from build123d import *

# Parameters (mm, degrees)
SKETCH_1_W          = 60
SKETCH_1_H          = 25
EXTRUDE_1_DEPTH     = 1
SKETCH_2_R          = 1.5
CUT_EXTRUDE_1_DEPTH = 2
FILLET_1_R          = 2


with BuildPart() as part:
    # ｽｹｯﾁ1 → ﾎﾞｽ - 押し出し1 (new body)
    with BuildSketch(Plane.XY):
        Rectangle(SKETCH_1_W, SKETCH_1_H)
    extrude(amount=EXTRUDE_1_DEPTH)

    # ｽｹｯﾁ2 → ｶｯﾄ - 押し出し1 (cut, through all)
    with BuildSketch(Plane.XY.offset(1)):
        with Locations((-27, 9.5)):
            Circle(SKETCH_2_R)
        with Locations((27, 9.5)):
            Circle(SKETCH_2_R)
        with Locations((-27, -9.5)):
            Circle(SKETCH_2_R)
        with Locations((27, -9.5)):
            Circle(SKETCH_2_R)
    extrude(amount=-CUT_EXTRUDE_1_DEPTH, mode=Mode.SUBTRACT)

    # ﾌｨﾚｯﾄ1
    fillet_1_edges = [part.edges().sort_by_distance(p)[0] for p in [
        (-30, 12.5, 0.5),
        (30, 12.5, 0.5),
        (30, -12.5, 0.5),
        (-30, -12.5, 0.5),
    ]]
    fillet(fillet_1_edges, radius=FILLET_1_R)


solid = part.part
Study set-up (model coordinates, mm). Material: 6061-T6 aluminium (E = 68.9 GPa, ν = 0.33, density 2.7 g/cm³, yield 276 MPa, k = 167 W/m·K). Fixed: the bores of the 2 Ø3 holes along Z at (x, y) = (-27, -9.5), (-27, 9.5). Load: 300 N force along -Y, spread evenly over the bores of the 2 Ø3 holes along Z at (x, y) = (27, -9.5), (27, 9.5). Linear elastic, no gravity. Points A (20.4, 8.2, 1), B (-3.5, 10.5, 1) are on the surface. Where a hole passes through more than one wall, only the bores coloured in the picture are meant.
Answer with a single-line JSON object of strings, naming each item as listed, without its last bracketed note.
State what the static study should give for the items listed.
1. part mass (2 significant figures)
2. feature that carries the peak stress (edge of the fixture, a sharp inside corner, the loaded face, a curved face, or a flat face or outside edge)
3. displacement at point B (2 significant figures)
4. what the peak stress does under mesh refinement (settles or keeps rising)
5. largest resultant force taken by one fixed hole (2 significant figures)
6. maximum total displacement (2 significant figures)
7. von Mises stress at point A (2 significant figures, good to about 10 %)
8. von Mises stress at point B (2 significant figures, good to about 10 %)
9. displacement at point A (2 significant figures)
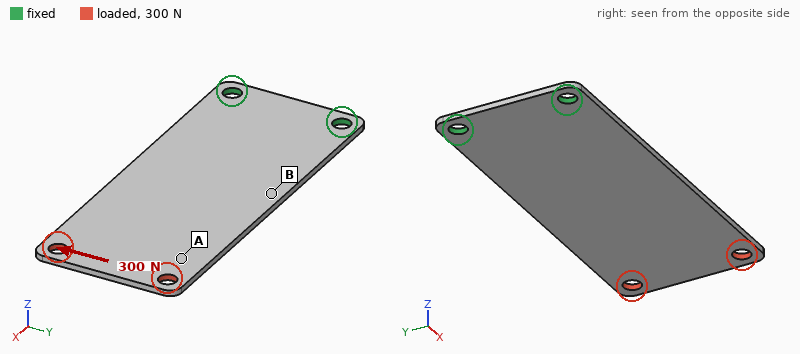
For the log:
{"part mass": "4.0 g", "feature that carries the peak stress": "edge of the fixture", "displacement at point B": "0.065 mm", "what the peak stress does under mesh refinement": "keeps rising", "largest resultant force taken by one fixed hole": "830 N", "maximum total displacement": "0.23 mm", "von Mises stress at point A": "22 MPa", "von Mises stress at point B": "74 MPa", "displacement at point A": "0.17 mm"}
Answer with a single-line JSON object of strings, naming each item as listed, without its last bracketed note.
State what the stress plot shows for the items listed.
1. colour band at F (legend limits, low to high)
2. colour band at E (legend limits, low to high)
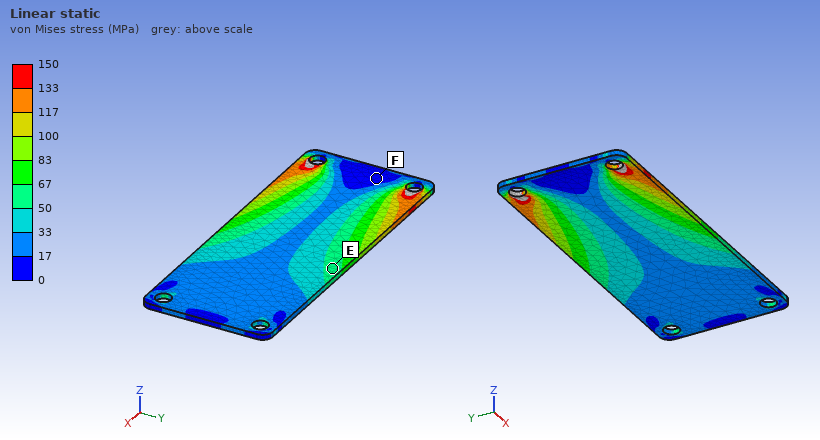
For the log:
{"colour band at F": "0 to 17 MPa", "colour band at E": "50 to 67 MPa"}
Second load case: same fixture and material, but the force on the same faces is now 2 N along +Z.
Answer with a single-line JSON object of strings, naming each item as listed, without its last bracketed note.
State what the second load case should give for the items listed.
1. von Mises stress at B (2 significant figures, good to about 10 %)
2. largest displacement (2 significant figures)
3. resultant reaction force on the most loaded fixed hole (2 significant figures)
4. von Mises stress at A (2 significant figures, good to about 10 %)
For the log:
{"von Mises stress at B": "15 MPa", "largest displacement": "0.77 mm", "resultant reaction force on the most loaded fixed hole": "1.0 N", "von Mises stress at A": "3.6 MPa"}
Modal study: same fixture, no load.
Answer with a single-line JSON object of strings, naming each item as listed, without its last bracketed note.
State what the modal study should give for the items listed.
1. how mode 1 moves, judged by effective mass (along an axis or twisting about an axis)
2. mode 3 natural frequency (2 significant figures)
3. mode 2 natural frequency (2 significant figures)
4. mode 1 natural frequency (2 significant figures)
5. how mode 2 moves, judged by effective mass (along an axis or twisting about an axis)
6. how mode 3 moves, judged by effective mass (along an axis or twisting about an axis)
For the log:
{"how mode 1 moves, judged by effective mass": "along Z", "mode 3 natural frequency": "1600 Hz", "mode 2 natural frequency": "1300 Hz", "mode 1 natural frequency": "260 Hz", "how mode 2 moves, judged by effective mass": "twisting about X", "how mode 3 moves, judged by effective mass": "along Z"}
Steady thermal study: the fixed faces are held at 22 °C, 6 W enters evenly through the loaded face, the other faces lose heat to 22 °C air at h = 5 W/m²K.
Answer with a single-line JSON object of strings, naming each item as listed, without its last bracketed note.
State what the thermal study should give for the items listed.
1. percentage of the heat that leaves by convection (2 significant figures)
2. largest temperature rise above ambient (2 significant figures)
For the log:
{"percentage of the heat that leaves by convection": "9.7 %", "largest temperature rise above ambient": "81 K"}
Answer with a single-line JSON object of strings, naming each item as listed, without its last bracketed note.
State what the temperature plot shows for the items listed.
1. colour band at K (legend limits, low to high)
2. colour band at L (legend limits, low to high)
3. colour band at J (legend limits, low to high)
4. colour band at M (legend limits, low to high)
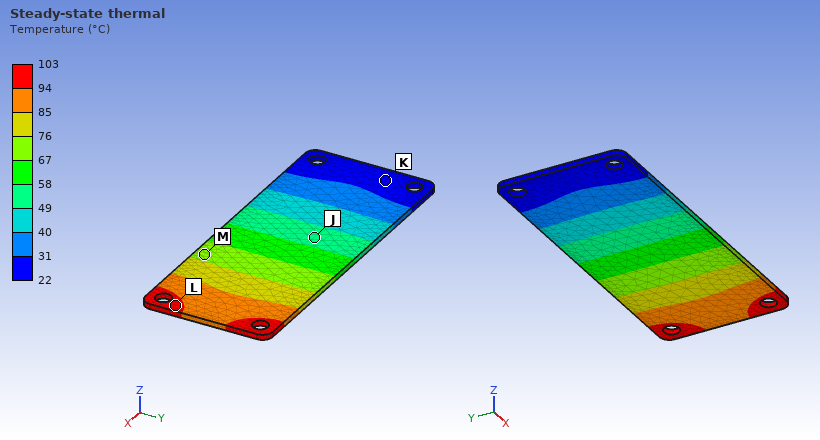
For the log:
{"colour band at K": "22 to 31 °C", "colour band at L": "94 to 103 °C", "colour band at J": "49 to 58 °C", "colour band at M": "67 to 76 °C"}
